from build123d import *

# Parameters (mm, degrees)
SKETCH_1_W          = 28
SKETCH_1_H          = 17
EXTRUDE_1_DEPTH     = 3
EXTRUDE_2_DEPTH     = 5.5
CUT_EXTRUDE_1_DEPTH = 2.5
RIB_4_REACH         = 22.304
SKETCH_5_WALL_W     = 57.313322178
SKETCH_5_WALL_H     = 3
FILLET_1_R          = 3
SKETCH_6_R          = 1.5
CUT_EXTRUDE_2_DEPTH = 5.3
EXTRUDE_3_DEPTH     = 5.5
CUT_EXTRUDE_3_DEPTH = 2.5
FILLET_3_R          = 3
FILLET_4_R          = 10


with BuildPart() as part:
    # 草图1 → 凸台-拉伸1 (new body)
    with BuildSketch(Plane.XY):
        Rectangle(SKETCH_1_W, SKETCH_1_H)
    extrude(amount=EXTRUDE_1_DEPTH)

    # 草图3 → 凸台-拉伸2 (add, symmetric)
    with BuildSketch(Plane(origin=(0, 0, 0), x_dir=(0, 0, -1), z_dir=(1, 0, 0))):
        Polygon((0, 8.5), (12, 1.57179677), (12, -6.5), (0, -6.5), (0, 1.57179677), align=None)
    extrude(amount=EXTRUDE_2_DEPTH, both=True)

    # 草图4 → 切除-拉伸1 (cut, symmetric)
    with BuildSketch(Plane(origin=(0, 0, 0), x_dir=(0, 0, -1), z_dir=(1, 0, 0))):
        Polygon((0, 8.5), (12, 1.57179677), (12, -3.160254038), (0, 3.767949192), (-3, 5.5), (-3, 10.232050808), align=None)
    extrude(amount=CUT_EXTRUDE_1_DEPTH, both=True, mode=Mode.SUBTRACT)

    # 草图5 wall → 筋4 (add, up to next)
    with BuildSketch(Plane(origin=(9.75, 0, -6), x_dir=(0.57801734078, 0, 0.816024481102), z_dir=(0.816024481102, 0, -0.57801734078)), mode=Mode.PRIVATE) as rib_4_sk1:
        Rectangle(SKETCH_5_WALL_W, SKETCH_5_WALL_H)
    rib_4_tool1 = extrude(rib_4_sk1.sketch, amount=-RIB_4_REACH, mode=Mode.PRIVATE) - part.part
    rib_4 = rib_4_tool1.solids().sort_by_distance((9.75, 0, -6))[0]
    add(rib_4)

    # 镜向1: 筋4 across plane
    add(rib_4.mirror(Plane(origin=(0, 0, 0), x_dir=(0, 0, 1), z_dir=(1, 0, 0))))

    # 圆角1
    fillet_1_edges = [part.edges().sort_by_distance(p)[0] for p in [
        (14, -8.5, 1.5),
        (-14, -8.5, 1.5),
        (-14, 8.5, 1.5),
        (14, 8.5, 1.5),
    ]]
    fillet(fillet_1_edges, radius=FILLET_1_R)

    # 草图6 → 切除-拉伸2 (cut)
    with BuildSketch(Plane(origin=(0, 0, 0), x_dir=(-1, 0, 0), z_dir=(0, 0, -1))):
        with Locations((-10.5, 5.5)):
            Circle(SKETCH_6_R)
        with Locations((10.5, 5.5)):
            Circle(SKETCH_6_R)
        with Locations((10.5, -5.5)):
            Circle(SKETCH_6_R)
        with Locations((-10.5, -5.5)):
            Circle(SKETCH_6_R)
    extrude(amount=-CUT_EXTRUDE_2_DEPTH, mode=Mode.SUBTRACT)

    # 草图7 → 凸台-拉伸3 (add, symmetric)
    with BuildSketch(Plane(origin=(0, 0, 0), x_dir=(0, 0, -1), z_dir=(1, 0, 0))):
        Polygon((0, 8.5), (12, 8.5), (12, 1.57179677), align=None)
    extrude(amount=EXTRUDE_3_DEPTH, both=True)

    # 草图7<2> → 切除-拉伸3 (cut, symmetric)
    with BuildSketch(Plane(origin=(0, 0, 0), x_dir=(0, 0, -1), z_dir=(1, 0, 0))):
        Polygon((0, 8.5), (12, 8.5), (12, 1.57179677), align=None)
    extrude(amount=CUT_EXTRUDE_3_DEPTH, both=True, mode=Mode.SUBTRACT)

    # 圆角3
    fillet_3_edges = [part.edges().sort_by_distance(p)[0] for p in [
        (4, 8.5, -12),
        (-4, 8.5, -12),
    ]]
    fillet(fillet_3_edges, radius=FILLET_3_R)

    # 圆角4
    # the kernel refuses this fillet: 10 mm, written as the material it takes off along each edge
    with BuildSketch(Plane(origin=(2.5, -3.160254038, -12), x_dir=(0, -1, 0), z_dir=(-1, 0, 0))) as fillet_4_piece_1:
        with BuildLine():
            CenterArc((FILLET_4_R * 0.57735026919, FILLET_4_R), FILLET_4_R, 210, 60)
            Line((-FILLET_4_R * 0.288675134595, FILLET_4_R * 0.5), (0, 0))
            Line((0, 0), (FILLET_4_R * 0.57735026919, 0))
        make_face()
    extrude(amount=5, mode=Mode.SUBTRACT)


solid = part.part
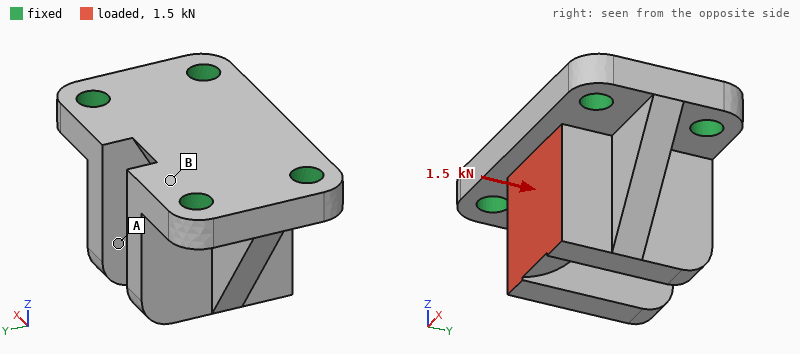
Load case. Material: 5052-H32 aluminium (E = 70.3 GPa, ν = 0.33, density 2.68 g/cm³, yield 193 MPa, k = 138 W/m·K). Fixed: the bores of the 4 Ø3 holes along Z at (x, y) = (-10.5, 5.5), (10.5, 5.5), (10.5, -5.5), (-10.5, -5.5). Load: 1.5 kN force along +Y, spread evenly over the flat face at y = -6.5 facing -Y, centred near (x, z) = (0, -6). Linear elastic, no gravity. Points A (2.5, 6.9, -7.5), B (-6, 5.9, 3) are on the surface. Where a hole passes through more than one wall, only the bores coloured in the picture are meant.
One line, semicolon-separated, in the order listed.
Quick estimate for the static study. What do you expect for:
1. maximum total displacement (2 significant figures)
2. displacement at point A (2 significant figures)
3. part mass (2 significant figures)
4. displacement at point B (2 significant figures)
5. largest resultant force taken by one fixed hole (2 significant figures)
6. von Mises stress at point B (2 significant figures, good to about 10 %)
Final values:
37 µm; 25 µm; 8.1 g; 7.4 µm; 720 N; 31 MPa
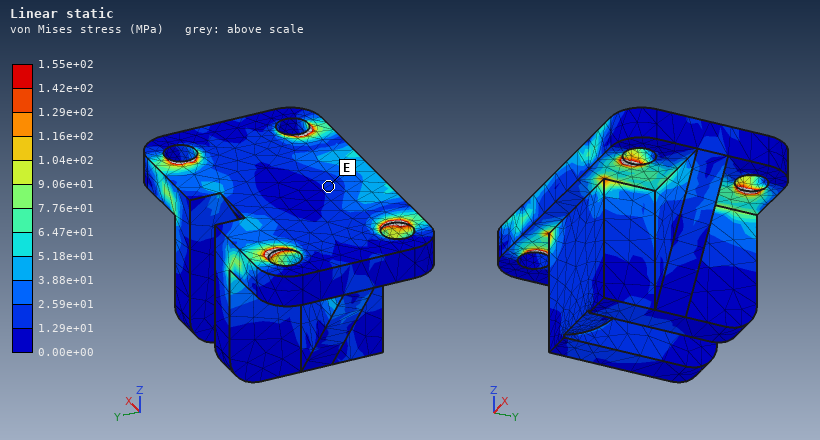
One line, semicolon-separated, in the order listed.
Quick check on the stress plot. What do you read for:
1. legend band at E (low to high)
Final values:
1.29e+01 to 2.59e+01 MPa
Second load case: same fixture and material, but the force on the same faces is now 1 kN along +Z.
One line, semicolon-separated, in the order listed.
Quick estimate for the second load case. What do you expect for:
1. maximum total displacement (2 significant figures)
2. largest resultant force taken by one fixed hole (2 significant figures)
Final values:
25 µm; 560 N
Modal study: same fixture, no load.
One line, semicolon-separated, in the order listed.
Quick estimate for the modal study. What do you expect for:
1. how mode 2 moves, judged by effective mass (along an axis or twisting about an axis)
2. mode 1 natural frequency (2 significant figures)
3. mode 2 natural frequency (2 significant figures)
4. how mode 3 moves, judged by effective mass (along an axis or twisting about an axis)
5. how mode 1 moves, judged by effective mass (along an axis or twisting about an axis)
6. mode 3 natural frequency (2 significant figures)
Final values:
along Z; 18 kHz; 28 kHz; along X; along Y; 30 kHz
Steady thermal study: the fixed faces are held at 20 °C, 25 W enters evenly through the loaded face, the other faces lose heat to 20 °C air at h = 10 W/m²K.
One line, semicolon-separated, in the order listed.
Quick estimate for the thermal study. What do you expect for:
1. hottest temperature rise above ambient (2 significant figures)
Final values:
24 K
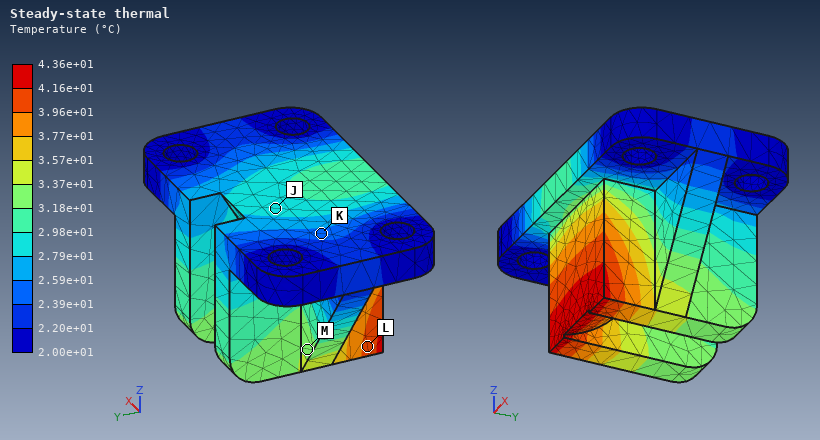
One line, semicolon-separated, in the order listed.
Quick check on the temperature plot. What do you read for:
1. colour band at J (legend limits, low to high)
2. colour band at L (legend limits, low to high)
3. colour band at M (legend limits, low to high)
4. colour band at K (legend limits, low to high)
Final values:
2.79e+01 to 2.98e+01 °C; 3.96e+01 to 4.16e+01 °C; 3.18e+01 to 3.37e+01 °C; 2.39e+01 to 2.59e+01 °C
